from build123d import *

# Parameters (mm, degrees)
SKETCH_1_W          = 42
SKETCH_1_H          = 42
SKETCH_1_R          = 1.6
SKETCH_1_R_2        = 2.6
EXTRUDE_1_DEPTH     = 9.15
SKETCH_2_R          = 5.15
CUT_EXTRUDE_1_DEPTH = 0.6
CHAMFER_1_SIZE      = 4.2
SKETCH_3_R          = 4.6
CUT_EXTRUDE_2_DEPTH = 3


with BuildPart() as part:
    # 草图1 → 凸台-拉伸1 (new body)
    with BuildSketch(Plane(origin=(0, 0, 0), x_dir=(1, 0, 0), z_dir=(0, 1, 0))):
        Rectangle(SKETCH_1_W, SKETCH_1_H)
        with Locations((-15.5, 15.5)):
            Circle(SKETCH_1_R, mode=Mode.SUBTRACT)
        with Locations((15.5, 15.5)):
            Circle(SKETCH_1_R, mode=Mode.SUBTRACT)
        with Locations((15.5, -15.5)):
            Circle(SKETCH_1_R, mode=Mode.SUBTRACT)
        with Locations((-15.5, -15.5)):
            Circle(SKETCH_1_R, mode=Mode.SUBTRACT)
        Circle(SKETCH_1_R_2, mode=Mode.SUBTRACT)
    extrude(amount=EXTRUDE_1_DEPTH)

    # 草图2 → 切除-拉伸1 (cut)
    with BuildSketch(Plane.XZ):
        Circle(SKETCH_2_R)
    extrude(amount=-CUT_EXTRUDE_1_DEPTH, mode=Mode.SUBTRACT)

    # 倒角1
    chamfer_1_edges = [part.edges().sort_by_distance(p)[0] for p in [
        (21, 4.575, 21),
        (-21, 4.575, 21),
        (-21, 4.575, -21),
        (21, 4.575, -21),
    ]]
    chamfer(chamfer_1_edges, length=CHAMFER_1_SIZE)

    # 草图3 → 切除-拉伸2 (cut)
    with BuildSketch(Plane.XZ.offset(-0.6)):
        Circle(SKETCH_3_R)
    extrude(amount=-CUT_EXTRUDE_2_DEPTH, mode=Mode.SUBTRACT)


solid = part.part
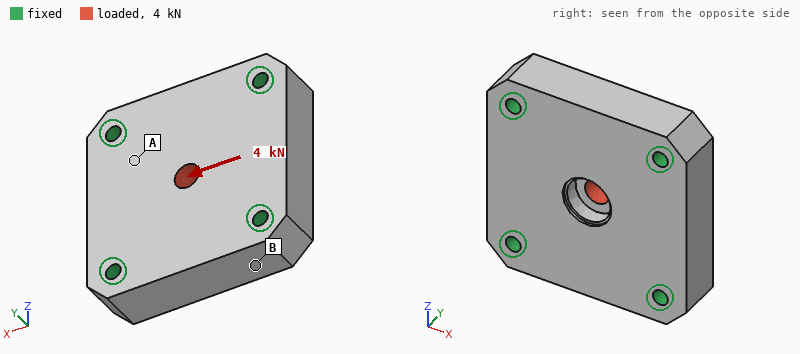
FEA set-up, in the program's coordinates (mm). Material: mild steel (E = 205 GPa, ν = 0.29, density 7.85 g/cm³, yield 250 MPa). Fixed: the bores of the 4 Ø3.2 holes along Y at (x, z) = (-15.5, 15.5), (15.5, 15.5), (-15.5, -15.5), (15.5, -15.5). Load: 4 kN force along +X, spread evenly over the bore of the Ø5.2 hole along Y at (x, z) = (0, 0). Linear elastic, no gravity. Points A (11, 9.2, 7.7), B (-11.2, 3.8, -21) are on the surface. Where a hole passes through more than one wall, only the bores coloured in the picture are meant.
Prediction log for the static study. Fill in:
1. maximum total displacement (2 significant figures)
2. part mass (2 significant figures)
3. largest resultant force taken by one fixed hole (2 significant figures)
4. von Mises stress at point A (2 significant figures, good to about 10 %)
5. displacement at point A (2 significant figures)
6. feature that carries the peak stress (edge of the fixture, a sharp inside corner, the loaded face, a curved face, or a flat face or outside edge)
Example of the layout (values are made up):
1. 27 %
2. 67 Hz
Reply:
1. 2.3 µm
2. 120 g
3. 1.1 kN
4. 15 MPa
5. 0.79 µm
6. the loaded face
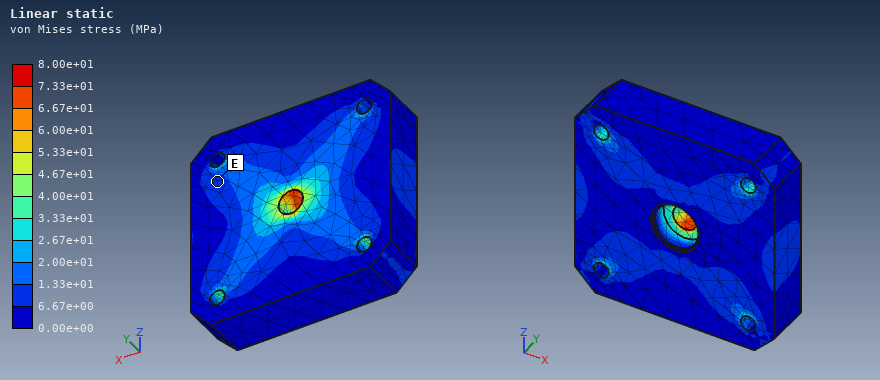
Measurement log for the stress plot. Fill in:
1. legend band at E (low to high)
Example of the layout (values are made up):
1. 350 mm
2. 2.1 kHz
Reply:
1. 6.67e+00 to 1.33e+01 MPa
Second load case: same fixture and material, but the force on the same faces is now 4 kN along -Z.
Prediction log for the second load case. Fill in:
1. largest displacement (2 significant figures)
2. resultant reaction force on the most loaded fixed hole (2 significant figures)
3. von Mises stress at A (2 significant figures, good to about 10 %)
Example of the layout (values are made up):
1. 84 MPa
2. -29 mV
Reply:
1. 2.3 µm
2. 1.1 kN
3. 13 MPa
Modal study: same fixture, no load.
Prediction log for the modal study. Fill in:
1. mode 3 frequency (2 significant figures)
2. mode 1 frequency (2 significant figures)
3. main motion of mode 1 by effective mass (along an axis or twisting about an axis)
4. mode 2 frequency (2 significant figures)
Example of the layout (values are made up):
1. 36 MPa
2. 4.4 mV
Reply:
1. 36 kHz
2. 25 kHz
3. along Y
4. 36 kHz
